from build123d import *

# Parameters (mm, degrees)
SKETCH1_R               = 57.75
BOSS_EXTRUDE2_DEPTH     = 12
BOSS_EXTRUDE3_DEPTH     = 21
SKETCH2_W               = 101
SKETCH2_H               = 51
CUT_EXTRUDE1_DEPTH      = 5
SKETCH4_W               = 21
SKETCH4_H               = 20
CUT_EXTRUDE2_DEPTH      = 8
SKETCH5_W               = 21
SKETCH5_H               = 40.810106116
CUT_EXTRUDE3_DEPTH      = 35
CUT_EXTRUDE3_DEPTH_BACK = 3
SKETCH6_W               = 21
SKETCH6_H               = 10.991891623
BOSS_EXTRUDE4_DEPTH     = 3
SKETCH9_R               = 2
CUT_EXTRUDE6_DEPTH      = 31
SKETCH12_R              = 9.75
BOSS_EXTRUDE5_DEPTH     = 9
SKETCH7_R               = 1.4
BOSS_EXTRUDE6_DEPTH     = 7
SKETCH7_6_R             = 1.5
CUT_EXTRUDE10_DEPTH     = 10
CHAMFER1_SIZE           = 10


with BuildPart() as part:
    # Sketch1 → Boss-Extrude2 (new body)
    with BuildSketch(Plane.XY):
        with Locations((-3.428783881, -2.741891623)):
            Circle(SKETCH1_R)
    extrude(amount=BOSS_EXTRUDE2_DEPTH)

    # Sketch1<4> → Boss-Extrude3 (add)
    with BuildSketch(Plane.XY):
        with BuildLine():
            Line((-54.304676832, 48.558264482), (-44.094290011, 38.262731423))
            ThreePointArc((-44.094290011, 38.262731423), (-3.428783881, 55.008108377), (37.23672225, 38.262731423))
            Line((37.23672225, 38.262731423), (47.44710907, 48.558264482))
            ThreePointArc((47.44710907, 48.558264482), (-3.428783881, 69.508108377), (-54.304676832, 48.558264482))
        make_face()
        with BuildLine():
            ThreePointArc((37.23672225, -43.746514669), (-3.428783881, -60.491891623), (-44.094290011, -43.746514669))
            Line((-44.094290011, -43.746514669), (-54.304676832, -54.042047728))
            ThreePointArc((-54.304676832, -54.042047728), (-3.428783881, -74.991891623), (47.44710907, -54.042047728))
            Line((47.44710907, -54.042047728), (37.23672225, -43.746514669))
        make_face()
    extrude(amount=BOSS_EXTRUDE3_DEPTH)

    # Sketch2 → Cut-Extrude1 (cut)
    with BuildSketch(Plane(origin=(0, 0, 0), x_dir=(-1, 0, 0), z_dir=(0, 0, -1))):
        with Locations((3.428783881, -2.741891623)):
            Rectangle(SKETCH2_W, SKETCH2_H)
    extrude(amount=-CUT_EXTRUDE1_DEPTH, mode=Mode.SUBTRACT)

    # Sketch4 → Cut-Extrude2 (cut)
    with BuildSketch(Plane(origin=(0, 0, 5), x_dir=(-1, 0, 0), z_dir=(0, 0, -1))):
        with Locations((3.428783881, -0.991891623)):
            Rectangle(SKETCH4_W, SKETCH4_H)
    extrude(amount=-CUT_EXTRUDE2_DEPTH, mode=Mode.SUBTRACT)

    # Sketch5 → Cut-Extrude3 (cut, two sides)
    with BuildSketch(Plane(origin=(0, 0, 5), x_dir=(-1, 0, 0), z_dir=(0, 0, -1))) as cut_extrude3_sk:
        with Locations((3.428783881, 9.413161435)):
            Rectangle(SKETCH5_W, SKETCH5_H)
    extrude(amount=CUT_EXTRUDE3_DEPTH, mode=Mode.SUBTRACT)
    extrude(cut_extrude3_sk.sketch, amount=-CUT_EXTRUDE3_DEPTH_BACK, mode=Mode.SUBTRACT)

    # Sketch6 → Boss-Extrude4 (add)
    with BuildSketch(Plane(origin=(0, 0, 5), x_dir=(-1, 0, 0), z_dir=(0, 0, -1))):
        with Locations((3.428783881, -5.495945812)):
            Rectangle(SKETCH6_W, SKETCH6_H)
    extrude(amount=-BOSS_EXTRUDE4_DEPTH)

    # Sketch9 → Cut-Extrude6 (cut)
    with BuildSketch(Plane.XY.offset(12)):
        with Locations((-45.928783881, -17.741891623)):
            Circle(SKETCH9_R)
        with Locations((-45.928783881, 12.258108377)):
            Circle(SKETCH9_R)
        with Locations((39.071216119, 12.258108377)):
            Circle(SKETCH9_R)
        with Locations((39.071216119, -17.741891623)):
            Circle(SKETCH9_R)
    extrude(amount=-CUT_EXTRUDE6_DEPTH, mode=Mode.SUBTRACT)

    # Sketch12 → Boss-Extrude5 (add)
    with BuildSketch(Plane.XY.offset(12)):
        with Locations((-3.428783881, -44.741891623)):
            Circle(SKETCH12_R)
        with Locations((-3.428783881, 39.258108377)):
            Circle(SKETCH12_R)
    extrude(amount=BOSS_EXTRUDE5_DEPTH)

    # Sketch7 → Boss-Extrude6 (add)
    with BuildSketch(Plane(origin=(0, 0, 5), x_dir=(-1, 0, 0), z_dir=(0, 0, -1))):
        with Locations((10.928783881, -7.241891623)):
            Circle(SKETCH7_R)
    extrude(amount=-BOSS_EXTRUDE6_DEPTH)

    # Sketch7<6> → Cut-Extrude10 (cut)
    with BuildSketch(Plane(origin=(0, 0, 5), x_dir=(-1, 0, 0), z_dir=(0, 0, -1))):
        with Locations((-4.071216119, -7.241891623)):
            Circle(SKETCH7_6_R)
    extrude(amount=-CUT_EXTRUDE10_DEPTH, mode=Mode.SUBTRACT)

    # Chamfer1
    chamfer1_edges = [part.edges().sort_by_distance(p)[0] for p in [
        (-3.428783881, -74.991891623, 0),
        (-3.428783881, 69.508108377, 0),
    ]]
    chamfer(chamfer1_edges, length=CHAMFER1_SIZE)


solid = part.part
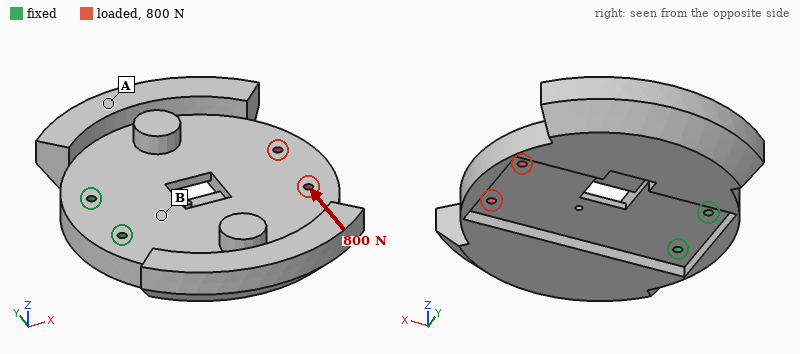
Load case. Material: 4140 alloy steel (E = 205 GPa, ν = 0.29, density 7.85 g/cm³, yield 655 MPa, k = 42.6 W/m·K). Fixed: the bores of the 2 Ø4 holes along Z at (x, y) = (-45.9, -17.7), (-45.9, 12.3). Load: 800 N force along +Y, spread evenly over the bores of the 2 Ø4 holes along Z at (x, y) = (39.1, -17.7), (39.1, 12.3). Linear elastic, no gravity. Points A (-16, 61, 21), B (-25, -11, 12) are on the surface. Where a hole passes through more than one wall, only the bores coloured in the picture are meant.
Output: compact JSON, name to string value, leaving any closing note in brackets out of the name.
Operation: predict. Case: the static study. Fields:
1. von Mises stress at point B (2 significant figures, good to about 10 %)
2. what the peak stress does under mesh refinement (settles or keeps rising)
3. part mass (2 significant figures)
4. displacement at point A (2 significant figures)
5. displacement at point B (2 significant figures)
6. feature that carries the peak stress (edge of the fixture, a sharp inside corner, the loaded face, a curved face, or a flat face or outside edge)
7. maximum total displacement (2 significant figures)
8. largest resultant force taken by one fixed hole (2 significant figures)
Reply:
{"von Mises stress at point B": "7.4 MPa", "what the peak stress does under mesh refinement": "keeps rising", "part mass": "1.2 kg", "displacement at point A": "8.4 µm", "displacement at point B": "2.5 µm", "feature that carries the peak stress": "edge of the fixture", "maximum total displacement": "14 µm", "largest resultant force taken by one fixed hole": "2.1 kN"}
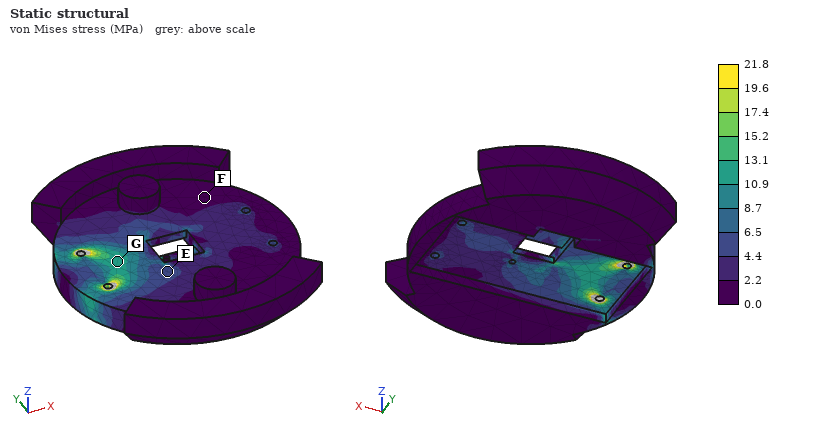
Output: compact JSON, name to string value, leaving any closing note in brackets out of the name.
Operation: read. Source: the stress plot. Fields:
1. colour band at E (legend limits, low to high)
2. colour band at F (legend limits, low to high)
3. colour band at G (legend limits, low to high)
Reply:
{"colour band at E": "4.4 to 6.5 MPa", "colour band at F": "0.0 to 2.2 MPa", "colour band at G": "10.9 to 13.1 MPa"}
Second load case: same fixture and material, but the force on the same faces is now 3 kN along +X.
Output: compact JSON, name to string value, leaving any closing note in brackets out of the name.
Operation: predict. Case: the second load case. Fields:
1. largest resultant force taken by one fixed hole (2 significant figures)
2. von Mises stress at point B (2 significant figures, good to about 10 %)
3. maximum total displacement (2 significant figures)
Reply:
{"largest resultant force taken by one fixed hole": "1.5 kN", "von Mises stress at point B": "7.8 MPa", "maximum total displacement": "6.3 µm"}
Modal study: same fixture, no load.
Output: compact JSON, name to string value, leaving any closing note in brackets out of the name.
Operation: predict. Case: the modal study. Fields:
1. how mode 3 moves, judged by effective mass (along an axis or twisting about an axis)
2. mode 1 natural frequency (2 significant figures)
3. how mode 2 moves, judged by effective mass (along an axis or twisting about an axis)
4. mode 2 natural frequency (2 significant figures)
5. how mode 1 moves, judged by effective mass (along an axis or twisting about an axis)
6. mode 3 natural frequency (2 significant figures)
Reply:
{"how mode 3 moves, judged by effective mass": "along Y", "mode 1 natural frequency": "490 Hz", "how mode 2 moves, judged by effective mass": "twisting about X", "mode 2 natural frequency": "710 Hz", "how mode 1 moves, judged by effective mass": "along Z", "mode 3 natural frequency": "1600 Hz"}
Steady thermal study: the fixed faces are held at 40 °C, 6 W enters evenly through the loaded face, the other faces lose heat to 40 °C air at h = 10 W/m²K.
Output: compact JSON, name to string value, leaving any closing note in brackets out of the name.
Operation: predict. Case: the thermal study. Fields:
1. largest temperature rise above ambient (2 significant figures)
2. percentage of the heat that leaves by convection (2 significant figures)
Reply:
{"largest temperature rise above ambient": "15 K", "percentage of the heat that leaves by convection": "40 %"}
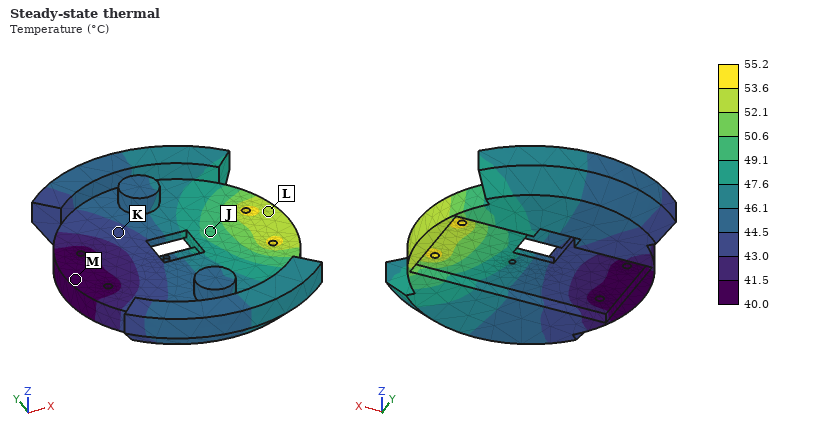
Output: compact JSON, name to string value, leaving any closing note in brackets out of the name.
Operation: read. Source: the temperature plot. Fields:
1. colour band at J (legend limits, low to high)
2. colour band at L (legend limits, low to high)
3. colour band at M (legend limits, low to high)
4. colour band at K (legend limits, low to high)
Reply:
{"colour band at J": "49.1 to 50.6 °C", "colour band at L": "52.1 to 53.6 °C", "colour band at M": "40.0 to 41.5 °C", "colour band at K": "43.0 to 44.5 °C"}
